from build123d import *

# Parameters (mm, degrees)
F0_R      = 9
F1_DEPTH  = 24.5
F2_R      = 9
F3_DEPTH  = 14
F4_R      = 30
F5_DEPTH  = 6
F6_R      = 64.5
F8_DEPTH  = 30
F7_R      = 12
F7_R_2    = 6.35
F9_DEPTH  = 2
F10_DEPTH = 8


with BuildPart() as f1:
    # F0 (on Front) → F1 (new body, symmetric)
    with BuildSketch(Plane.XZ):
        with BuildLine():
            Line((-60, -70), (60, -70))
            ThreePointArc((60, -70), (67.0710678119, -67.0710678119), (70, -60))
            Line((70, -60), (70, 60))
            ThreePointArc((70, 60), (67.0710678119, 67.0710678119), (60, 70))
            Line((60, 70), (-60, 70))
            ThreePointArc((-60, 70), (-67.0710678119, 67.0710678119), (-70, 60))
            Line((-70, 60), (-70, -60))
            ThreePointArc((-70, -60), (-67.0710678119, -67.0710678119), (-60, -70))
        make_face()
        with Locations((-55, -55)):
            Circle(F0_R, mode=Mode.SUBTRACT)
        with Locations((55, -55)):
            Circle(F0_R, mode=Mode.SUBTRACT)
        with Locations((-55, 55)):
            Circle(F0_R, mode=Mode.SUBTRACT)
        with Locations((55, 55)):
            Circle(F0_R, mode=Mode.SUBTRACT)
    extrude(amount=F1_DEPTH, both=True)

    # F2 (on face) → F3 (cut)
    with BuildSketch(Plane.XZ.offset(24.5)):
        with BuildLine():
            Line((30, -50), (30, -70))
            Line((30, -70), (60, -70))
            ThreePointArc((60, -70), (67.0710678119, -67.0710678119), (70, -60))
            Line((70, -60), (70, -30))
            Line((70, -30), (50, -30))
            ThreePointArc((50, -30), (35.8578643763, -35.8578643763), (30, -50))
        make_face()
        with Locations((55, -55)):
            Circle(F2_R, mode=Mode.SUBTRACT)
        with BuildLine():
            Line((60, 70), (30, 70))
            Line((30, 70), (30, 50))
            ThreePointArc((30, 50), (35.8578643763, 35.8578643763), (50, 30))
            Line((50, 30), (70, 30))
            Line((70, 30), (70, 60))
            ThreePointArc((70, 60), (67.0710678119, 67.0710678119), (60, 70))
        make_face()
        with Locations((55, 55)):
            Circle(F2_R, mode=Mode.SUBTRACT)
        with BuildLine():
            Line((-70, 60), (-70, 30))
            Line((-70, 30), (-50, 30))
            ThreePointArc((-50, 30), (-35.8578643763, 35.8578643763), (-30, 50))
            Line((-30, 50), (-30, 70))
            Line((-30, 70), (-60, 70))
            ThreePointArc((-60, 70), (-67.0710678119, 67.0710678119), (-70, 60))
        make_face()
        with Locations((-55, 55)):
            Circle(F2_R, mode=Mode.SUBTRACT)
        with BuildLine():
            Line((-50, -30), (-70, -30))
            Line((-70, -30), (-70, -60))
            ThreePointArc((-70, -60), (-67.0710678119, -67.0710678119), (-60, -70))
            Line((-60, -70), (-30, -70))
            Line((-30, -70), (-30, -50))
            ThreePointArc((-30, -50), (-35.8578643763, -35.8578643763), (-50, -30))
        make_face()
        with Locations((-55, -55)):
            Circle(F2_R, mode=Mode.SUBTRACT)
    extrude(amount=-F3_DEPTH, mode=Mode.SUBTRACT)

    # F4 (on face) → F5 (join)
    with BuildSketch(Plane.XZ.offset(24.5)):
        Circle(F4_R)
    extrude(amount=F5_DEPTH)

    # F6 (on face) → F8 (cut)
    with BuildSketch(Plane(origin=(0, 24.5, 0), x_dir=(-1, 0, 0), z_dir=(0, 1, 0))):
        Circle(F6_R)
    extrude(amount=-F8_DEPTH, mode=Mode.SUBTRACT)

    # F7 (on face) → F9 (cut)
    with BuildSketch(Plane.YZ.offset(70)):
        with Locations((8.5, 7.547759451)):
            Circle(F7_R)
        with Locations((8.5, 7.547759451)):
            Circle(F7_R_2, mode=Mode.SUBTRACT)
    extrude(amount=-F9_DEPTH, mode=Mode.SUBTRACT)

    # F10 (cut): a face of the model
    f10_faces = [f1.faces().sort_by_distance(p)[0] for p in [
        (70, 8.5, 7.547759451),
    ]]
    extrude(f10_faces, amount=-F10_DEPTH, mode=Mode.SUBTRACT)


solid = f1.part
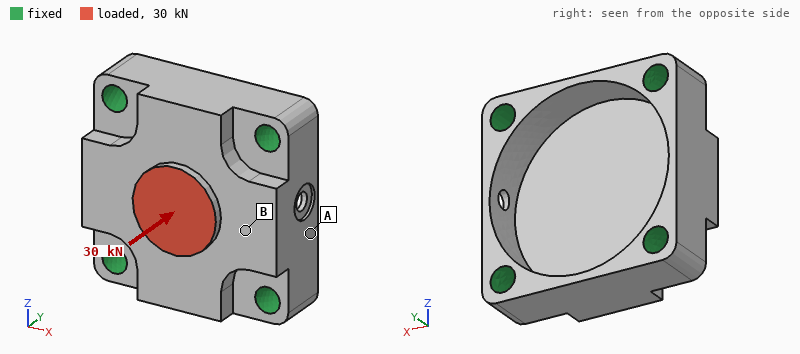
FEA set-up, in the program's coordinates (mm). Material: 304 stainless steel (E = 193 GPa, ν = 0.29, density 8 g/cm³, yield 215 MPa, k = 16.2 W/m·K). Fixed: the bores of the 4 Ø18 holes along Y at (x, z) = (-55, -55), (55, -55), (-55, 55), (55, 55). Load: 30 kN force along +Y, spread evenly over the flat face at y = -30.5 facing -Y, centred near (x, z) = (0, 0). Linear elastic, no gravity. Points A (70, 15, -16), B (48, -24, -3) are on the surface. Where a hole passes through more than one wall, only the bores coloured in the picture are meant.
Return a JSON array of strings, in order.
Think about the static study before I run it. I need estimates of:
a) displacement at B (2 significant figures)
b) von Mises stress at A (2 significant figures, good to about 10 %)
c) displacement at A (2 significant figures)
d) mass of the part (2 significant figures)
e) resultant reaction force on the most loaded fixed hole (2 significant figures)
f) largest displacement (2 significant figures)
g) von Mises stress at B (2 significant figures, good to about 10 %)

["13 µm", "7.7 MPa", "4.3 µm", "3.7 kg", "11 kN", "28 µm", "18 MPa"]
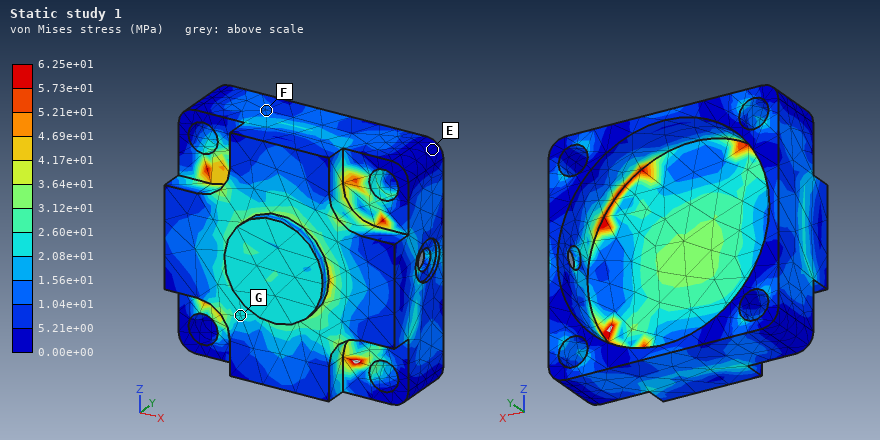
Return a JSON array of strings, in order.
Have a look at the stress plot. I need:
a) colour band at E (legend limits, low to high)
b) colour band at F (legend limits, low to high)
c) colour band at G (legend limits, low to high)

["0.00e+00 to 5.21e+00 MPa", "1.04e+01 to 1.56e+01 MPa", "2.08e+01 to 2.60e+01 MPa"]
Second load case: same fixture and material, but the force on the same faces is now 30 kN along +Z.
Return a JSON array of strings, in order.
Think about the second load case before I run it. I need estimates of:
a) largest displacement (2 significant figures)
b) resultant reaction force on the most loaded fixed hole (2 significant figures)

["11 µm", "9.0 kN"]
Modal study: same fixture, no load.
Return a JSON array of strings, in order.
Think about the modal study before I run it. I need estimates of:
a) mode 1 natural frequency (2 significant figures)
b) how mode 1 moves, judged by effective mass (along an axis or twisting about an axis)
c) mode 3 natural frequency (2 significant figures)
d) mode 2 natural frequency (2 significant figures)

["5300 Hz", "along Y", "8700 Hz", "8600 Hz"]
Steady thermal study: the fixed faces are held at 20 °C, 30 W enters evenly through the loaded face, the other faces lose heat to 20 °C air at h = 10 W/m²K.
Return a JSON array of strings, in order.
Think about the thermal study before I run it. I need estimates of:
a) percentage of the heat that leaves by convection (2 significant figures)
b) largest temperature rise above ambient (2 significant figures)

["22 %", "35 K"]
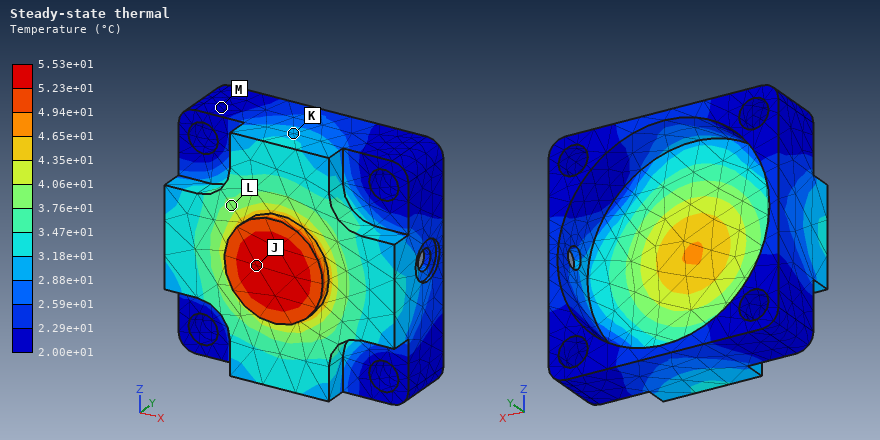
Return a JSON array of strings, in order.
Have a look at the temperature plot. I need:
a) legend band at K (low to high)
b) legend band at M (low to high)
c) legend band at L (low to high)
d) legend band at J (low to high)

["2.88e+01 to 3.18e+01 °C", "2.00e+01 to 2.29e+01 °C", "3.76e+01 to 4.06e+01 °C", "5.23e+01 to 5.53e+01 °C"]
